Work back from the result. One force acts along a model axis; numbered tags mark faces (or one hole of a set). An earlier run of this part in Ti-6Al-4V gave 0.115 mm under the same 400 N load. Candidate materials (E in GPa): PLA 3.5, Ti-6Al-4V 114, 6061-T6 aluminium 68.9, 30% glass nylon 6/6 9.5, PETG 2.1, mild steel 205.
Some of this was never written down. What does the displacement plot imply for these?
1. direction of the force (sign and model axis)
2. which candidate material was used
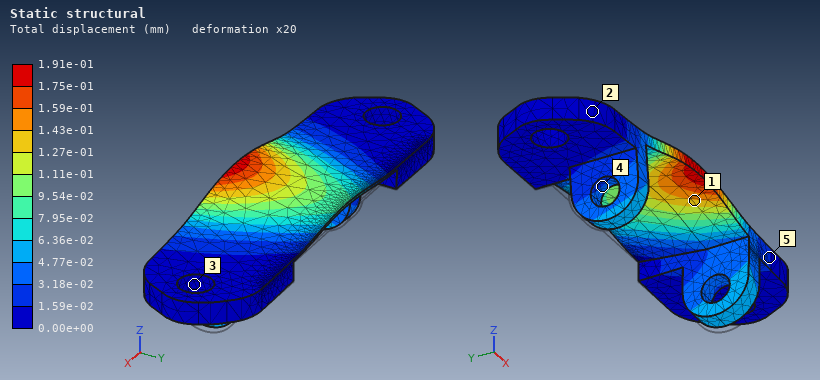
+Z
6061-T6 aluminium
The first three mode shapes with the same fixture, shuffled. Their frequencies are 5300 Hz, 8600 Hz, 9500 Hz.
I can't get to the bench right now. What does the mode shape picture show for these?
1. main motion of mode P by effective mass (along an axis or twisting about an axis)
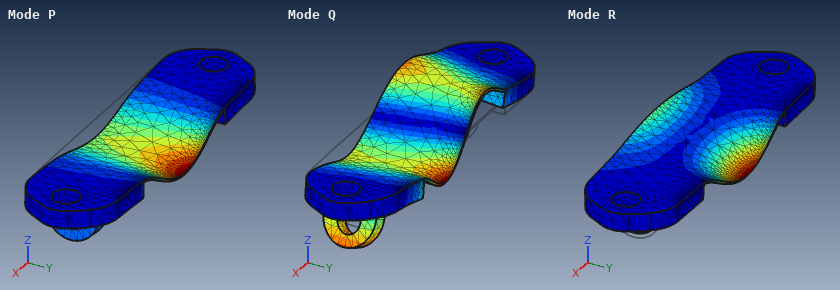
along Z
